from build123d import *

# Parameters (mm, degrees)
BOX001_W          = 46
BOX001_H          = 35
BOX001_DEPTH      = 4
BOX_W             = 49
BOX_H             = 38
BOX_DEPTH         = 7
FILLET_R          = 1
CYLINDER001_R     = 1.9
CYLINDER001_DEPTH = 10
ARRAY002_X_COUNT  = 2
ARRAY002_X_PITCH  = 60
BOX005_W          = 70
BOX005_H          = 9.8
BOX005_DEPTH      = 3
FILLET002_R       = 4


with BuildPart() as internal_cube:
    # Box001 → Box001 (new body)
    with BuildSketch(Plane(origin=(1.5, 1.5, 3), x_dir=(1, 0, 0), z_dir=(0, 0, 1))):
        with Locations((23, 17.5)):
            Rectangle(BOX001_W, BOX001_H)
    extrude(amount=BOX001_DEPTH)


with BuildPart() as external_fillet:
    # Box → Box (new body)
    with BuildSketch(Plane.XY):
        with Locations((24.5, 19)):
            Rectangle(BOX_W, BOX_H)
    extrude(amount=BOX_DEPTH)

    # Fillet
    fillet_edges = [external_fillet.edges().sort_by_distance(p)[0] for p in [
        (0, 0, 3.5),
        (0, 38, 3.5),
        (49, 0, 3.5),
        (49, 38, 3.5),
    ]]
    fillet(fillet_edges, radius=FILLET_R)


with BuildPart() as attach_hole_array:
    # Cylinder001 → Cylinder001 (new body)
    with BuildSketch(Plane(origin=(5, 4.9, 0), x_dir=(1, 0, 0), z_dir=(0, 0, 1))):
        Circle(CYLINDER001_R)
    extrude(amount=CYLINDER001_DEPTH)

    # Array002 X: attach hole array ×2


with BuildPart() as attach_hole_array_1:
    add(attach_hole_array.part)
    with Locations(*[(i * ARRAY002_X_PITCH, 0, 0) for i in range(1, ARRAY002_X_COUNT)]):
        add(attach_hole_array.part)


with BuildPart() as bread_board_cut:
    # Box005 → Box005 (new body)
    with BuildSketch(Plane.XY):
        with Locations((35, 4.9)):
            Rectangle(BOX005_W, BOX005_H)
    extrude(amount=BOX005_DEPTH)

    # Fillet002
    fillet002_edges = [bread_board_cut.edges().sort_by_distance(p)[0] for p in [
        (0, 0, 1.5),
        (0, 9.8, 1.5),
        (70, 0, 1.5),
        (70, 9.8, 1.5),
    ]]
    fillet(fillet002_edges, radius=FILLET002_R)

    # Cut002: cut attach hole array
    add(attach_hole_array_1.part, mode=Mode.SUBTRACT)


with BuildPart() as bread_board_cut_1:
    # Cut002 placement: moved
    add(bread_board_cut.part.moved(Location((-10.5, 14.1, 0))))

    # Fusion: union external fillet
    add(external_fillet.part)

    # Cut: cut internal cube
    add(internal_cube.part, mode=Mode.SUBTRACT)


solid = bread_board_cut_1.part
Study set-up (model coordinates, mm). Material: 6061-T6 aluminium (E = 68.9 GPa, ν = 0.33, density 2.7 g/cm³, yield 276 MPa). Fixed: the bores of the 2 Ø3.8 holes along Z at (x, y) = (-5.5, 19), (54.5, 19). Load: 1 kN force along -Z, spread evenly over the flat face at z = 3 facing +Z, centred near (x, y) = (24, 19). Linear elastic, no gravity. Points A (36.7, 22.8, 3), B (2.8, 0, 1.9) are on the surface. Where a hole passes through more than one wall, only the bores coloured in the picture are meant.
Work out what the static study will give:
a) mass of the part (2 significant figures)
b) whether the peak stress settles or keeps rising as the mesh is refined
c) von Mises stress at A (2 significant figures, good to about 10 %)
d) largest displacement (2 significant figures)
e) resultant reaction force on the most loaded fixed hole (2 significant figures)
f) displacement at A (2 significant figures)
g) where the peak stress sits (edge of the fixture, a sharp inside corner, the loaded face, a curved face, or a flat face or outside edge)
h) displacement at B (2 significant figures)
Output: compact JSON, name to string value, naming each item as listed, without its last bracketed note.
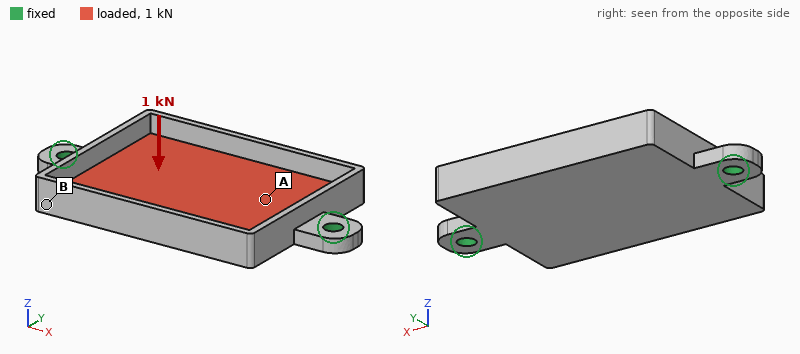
{"mass of the part": "19 g", "whether the peak stress settles or keeps rising as the mesh is refined": "keeps rising", "von Mises stress at A": "38 MPa", "largest displacement": "0.14 mm", "resultant reaction force on the most loaded fixed hole": "500 N", "displacement at A": "0.10 mm", "where the peak stress sits": "edge of the fixture", "displacement at B": "0.078 mm"}
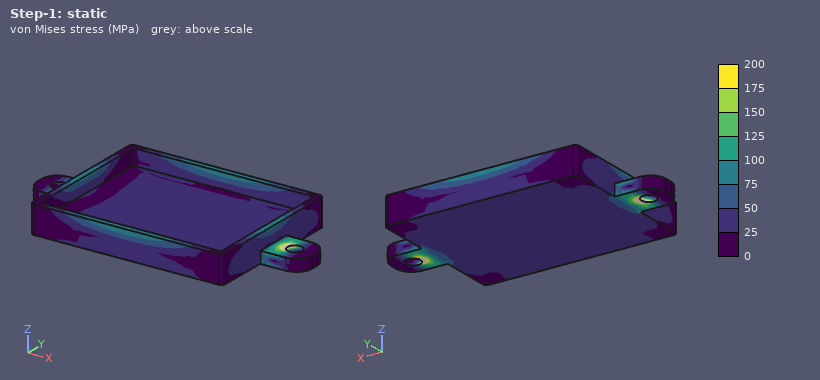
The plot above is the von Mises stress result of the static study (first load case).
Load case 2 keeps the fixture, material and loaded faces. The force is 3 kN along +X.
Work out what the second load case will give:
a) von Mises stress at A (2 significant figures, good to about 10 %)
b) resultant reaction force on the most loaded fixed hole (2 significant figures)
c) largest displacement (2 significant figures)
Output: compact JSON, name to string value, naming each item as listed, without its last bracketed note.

{"von Mises stress at A": "21 MPa", "resultant reaction force on the most loaded fixed hole": "1.5 kN", "largest displacement": "15 µm"}
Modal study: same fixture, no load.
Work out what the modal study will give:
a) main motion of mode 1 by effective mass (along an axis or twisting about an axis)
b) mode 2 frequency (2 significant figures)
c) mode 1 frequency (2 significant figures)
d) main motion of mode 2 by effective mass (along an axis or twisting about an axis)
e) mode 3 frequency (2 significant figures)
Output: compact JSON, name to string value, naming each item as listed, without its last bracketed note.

{"main motion of mode 1 by effective mass": "twisting about X", "mode 2 frequency": "3700 Hz", "mode 1 frequency": "2600 Hz", "main motion of mode 2 by effective mass": "along Z", "mode 3 frequency": "6300 Hz"}
